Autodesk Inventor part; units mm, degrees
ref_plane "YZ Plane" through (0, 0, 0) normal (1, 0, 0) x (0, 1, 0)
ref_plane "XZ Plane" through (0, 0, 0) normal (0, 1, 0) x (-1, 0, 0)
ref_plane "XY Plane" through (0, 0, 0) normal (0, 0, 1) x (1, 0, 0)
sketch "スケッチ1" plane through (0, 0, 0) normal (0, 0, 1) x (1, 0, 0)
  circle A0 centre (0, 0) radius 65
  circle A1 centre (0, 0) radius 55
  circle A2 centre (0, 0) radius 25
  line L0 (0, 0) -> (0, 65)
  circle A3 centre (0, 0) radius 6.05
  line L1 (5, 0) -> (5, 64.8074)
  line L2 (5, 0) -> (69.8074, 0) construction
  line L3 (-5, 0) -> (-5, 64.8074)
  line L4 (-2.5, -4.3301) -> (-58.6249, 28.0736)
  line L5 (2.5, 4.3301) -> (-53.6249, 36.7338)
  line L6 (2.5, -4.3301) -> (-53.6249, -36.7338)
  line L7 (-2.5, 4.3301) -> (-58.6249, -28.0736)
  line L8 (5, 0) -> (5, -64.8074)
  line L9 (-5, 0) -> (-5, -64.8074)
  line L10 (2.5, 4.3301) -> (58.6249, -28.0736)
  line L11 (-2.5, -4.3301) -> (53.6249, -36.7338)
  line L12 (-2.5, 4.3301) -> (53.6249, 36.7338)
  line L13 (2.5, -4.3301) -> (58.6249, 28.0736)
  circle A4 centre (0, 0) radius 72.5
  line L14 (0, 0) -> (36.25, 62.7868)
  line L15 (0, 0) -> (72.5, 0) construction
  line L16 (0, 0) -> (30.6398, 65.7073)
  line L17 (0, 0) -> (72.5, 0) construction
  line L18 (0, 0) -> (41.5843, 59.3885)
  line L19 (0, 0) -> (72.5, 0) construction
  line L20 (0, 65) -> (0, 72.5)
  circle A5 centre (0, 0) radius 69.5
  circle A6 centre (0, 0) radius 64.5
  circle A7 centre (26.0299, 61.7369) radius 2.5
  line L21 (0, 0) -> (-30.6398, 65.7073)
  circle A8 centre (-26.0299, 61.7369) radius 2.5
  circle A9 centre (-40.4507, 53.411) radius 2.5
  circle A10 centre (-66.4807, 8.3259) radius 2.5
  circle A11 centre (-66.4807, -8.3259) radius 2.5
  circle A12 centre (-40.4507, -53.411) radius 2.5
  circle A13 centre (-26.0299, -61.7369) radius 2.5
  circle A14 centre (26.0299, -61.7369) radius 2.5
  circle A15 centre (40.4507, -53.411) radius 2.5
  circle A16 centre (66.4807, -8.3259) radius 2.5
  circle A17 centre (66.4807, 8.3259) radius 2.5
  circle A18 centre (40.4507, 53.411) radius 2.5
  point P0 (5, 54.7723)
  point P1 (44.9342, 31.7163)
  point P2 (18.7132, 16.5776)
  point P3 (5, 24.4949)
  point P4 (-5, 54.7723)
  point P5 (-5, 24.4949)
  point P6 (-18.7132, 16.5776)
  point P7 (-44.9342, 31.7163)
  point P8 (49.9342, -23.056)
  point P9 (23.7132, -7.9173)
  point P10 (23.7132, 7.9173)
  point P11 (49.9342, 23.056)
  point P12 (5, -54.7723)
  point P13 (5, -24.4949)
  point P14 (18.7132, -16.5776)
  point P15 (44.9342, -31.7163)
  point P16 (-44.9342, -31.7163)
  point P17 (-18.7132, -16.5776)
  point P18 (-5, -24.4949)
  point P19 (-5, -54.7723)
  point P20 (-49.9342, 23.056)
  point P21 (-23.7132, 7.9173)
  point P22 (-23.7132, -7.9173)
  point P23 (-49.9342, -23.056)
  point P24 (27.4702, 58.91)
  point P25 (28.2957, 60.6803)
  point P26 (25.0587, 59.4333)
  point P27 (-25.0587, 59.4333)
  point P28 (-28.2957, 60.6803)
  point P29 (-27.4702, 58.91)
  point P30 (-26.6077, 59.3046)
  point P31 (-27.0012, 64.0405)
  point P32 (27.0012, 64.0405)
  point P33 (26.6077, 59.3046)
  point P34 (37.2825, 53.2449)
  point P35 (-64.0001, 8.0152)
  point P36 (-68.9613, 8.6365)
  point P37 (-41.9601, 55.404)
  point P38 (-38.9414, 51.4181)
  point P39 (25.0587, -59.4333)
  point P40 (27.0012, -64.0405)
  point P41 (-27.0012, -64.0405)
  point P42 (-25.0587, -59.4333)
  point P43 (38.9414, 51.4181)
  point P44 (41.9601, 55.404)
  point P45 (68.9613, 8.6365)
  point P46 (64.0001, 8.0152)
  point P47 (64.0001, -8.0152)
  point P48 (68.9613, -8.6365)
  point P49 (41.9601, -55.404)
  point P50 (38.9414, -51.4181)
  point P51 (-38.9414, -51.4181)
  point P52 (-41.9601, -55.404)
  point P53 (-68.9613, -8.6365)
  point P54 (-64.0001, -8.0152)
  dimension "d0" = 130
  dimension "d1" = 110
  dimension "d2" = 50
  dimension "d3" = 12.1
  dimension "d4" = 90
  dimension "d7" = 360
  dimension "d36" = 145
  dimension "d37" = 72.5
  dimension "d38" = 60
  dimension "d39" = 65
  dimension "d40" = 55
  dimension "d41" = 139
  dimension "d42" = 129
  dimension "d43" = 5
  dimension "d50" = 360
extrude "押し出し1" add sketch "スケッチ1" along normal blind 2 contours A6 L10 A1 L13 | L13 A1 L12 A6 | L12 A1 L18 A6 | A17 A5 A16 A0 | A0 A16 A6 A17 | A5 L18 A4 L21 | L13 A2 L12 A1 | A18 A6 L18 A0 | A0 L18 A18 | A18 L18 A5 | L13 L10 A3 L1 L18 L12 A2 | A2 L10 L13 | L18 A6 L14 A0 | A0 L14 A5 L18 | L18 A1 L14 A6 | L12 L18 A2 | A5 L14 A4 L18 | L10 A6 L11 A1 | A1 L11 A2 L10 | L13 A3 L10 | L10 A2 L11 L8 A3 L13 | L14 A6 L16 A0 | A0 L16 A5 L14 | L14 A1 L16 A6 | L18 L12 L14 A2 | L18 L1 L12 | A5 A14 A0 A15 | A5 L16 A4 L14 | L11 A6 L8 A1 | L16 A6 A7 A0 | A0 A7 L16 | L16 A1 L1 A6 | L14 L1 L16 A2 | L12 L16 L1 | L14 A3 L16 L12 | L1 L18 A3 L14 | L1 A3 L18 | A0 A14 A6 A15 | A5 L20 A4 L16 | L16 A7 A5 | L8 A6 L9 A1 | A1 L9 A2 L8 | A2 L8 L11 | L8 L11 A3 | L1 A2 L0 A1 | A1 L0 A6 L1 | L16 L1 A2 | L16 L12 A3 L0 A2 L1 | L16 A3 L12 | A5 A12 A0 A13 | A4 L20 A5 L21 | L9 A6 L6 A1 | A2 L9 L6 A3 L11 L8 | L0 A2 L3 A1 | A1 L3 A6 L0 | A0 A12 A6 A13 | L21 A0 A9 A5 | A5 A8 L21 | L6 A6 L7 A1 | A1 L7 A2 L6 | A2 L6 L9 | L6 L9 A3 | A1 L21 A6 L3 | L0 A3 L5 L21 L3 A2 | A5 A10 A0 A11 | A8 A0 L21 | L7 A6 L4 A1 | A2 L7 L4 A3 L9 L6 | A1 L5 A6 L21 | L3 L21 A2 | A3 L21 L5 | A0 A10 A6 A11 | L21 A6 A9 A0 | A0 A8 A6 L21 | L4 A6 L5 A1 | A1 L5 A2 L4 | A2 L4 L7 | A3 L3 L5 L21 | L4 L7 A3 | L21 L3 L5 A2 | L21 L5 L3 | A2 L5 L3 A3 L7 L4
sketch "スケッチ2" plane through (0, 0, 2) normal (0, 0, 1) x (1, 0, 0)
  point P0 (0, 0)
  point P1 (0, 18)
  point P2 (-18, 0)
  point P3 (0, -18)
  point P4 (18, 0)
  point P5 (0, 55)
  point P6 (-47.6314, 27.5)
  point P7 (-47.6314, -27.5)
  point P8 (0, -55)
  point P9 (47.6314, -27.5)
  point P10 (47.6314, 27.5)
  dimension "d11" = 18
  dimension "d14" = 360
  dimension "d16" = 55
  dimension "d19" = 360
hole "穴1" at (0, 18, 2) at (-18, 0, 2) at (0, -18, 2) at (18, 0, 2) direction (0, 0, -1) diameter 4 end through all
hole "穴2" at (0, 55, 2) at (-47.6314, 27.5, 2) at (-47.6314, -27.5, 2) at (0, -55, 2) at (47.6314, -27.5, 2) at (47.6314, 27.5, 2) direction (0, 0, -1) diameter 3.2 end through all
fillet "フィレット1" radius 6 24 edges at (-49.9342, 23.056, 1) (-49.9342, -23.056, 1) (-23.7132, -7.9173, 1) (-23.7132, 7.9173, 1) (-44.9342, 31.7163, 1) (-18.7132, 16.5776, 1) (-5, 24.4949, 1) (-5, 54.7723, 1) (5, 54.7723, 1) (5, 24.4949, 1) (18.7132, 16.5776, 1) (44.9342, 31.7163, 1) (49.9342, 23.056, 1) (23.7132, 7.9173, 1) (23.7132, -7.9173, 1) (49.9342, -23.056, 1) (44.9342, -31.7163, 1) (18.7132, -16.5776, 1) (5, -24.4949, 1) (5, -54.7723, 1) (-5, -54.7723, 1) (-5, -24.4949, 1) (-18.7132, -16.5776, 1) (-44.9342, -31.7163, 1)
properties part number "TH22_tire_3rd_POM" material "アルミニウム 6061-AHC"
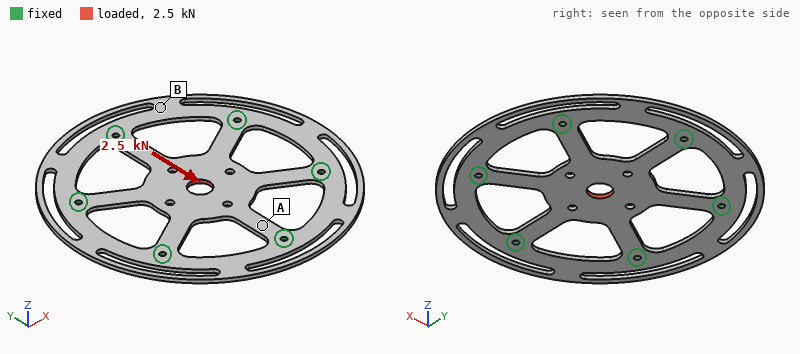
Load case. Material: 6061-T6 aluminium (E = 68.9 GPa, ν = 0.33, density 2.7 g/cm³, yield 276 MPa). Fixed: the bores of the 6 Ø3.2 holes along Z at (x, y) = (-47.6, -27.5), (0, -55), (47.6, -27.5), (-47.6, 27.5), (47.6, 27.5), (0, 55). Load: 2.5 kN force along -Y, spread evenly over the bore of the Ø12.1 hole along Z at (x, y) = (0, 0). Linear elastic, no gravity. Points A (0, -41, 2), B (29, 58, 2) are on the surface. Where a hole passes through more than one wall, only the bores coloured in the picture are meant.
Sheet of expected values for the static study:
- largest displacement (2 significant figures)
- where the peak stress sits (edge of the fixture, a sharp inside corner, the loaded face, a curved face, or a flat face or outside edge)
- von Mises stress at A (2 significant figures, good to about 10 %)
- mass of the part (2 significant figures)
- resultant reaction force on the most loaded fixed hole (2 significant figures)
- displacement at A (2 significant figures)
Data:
26 µm
a curved face
39 MPa
49 g
740 N
7.8 µm
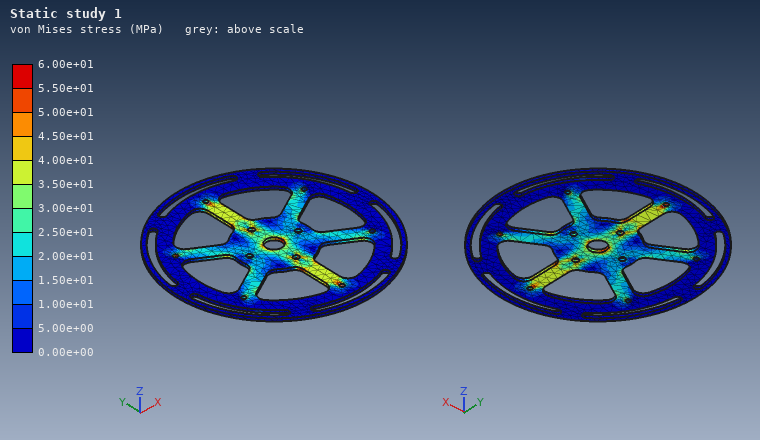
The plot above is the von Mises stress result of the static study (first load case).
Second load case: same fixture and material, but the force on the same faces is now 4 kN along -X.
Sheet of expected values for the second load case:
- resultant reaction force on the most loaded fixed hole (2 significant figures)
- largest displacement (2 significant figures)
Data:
1.0 kN
40 µm
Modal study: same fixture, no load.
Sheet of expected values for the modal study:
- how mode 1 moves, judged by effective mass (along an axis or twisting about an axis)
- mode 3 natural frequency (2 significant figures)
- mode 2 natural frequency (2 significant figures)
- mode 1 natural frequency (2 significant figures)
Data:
along Z
1400 Hz
1400 Hz
1100 Hz
